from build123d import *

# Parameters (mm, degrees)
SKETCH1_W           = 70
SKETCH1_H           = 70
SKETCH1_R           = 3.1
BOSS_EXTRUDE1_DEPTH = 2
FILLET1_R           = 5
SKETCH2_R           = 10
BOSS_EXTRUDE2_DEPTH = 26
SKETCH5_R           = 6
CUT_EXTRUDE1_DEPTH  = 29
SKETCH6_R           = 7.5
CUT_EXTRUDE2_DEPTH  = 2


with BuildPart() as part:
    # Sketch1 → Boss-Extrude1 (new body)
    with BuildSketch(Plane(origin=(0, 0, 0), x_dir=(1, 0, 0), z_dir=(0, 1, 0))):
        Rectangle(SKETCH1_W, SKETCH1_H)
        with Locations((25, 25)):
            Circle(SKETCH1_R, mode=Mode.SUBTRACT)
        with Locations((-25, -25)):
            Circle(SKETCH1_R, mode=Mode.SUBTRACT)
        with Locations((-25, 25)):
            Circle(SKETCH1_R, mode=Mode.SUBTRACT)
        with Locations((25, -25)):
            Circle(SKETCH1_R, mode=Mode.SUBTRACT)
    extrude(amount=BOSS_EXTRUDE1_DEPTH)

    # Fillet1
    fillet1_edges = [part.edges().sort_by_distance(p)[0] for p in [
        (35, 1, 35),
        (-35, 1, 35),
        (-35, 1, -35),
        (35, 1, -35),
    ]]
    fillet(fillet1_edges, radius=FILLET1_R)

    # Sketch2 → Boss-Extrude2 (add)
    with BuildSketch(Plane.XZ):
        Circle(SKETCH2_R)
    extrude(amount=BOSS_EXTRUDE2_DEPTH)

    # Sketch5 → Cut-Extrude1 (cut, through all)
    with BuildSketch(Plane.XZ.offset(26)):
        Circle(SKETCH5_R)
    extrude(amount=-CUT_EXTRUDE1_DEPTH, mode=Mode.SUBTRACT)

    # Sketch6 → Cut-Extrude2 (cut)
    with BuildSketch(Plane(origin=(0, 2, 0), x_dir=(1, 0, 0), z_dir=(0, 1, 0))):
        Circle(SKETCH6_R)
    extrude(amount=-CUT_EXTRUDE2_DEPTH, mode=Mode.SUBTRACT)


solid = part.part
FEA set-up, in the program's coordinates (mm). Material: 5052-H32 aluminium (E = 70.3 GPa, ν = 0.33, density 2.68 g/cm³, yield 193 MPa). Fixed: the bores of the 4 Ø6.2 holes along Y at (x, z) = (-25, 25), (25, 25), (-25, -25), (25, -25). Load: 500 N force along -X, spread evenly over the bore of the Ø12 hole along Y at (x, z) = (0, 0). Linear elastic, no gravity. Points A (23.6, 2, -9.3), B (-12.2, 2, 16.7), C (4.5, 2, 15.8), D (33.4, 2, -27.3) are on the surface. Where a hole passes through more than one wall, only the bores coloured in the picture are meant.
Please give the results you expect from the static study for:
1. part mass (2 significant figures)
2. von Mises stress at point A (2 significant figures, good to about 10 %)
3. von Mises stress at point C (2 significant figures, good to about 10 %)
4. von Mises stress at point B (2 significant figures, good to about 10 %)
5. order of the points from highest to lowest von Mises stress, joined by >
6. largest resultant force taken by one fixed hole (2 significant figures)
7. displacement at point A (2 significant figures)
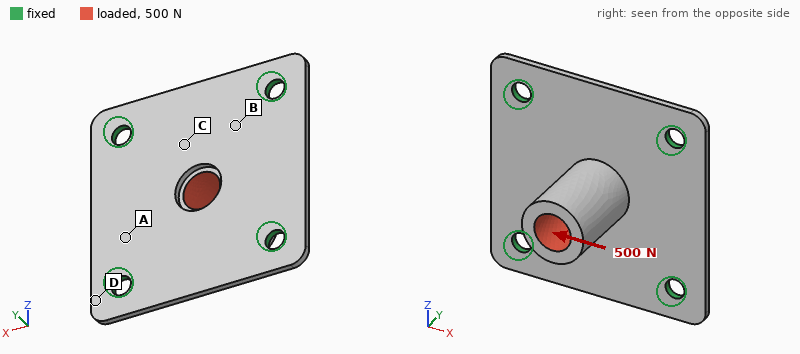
39 g
17 MPa
36 MPa
25 MPa
C > B > A > D
170 N
0.037 mm
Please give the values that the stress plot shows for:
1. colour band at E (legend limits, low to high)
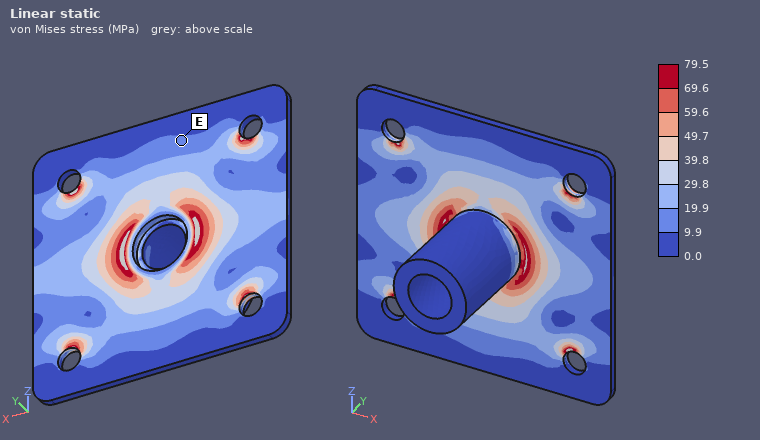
9.9 to 19.9 MPa
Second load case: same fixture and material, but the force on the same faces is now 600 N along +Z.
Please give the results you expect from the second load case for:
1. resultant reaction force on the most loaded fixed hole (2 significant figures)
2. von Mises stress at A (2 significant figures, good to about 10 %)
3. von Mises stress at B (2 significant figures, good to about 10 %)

200 N
21 MPa
21 MPa
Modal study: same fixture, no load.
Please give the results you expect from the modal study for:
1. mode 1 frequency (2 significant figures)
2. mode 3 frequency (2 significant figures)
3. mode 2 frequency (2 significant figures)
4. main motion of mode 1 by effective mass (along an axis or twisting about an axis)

2200 Hz
2400 Hz
2400 Hz
along Y
